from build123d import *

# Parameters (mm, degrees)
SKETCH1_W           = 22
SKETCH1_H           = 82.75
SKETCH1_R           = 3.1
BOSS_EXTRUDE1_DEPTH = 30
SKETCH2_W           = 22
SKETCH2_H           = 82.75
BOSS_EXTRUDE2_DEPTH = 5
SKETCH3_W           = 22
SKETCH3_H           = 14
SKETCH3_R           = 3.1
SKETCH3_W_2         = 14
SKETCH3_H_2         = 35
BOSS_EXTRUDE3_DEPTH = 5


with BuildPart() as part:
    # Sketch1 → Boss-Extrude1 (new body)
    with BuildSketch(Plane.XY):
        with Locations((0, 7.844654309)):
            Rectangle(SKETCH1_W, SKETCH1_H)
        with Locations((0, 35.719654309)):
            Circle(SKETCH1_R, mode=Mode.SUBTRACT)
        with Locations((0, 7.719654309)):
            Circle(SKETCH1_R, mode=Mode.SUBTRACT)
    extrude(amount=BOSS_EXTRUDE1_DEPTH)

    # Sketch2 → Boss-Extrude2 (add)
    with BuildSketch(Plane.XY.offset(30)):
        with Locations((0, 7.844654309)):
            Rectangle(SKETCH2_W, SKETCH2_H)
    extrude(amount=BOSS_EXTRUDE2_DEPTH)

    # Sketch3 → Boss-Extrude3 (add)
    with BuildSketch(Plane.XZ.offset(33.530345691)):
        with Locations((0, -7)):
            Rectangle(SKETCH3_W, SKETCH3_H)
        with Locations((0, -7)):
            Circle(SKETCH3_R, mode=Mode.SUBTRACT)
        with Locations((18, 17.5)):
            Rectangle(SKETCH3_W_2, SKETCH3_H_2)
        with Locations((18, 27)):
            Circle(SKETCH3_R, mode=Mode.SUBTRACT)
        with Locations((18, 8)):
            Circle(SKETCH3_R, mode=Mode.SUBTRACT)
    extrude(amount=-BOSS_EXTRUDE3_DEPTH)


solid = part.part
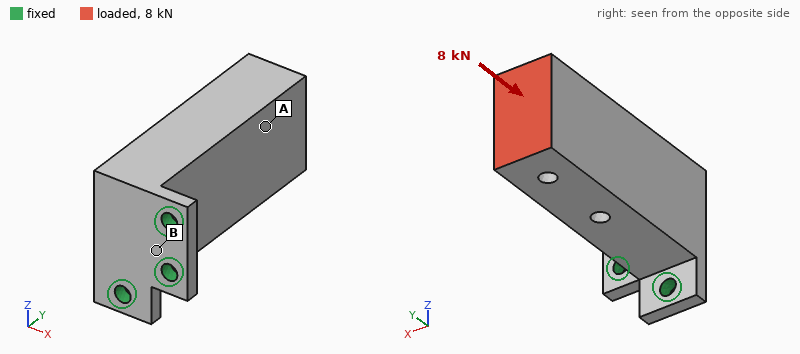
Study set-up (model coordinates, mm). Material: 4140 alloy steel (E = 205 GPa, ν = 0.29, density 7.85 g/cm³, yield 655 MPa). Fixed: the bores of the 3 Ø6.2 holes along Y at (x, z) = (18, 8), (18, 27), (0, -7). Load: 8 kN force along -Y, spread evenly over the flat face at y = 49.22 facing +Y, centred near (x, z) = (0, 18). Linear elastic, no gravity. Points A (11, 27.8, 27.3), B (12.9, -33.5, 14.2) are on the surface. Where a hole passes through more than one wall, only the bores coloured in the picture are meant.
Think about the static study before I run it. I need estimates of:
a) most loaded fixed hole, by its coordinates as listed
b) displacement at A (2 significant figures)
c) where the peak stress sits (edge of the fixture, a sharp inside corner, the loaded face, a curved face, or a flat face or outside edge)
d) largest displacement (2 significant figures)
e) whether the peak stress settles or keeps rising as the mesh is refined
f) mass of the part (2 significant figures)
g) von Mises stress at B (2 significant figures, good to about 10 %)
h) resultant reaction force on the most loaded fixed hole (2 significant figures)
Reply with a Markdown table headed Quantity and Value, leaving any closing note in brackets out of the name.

| Quantity | Value |
|---|---|
| most loaded fixed hole, by its coordinates as listed | (18, 27) |
| displacement at A | 0.15 mm |
| where the peak stress sits | edge of the fixture |
| largest displacement | 0.21 mm |
| whether the peak stress settles or keeps rising as the mesh is refined | keeps rising |
| mass of the part | 510 g |
| von Mises stress at B | 100 MPa |
| resultant reaction force on the most loaded fixed hole | 5.4 kN |
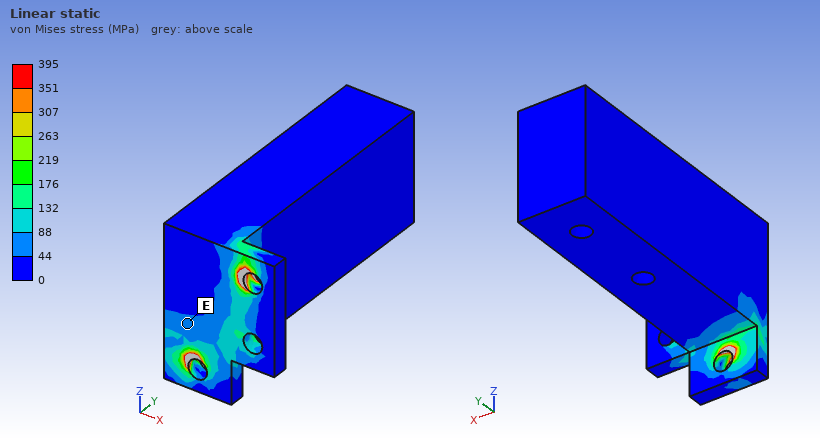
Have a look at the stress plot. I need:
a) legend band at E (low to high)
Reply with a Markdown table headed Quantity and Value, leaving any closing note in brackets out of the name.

| Quantity | Value |
|---|---|
| legend band at E | 44 to 88 MPa |
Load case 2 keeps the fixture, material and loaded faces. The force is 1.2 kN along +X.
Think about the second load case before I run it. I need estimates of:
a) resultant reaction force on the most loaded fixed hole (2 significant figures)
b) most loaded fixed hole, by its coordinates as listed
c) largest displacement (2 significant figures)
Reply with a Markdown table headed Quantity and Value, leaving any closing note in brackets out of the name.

| Quantity | Value |
|---|---|
| resultant reaction force on the most loaded fixed hole | 5.0 kN |
| most loaded fixed hole, by its coordinates as listed | (18, 8) |
| largest displacement | 0.25 mm |
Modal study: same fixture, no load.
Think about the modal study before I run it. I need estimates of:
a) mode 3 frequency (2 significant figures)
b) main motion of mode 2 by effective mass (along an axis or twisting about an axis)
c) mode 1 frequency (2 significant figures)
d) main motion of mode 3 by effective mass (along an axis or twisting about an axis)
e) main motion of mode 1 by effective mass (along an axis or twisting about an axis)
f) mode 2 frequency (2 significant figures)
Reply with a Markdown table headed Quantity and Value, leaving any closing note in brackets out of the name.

| Quantity | Value |
|---|---|
| mode 3 frequency | 6700 Hz |
| main motion of mode 2 by effective mass | along Z |
| mode 1 frequency | 860 Hz |
| main motion of mode 3 by effective mass | along Y |
| main motion of mode 1 by effective mass | along X |
| mode 2 frequency | 2000 Hz |
